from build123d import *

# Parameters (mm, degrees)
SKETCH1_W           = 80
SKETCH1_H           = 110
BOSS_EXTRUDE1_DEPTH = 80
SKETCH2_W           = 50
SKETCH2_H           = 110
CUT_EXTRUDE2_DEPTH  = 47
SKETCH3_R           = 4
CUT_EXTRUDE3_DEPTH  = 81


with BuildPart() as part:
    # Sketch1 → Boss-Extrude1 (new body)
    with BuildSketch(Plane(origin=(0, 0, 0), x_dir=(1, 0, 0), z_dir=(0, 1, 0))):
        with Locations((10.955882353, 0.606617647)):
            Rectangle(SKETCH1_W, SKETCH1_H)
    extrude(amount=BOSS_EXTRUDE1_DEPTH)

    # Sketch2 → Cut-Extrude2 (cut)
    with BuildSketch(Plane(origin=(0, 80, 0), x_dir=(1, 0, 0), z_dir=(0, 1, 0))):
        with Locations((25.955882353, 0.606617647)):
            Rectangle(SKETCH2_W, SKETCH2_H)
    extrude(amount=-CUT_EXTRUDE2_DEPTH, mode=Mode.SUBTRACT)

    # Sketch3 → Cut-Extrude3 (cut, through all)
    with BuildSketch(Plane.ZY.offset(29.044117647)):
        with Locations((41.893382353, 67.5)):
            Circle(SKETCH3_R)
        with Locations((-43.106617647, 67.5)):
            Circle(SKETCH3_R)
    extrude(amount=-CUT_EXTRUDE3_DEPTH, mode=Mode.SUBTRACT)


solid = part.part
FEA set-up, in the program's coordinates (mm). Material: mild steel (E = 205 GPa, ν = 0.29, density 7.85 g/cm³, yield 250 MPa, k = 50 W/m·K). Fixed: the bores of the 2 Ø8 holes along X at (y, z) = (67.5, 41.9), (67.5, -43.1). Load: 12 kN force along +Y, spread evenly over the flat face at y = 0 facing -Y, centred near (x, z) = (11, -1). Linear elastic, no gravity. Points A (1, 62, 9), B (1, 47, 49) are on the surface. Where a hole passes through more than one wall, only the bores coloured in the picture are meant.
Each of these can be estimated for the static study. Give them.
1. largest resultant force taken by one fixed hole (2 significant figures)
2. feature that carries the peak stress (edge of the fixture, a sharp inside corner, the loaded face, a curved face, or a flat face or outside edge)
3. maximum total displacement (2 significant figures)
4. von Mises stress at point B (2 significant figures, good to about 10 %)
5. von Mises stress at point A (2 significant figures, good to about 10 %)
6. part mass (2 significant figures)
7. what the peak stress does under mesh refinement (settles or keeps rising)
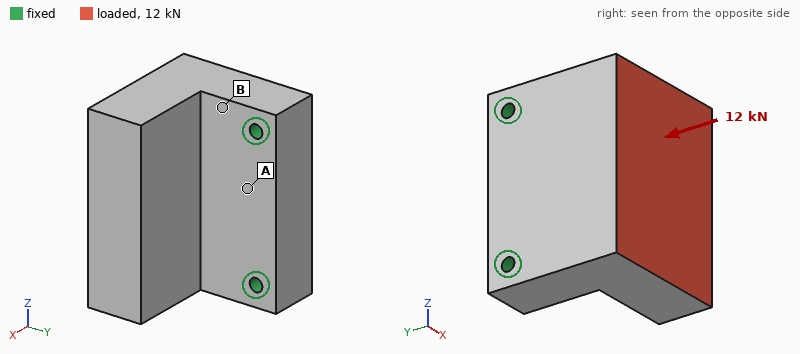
6.2 kN
edge of the fixture
34 µm
28 MPa
7.2 MPa
3.5 kg
keeps rising
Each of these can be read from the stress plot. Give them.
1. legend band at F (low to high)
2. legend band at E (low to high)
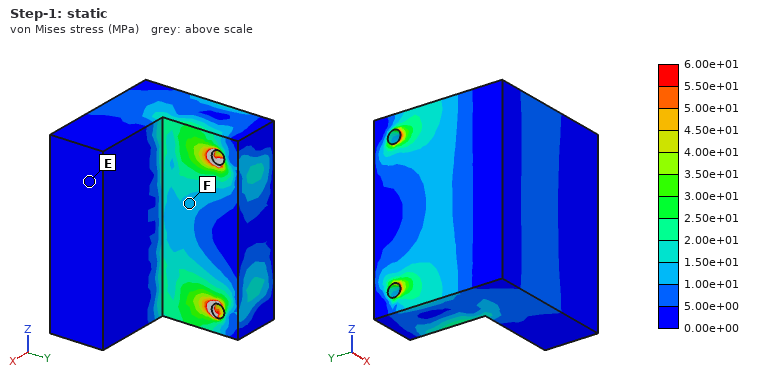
1.00e+01 to 1.50e+01 MPa
0.00e+00 to 5.00e+00 MPa
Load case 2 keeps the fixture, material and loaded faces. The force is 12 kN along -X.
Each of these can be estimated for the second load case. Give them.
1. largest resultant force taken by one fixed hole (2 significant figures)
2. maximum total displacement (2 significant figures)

6.0 kN
68 µm
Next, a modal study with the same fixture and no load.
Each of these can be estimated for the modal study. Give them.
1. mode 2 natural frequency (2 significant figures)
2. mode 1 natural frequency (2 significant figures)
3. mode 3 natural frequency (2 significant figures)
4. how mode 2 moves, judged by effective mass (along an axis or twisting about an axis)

3500 Hz
1800 Hz
5500 Hz
along Z
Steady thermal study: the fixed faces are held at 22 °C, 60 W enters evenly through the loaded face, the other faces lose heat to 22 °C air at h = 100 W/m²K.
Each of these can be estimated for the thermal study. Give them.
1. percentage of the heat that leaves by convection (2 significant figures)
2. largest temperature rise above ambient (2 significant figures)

50 %
17 K
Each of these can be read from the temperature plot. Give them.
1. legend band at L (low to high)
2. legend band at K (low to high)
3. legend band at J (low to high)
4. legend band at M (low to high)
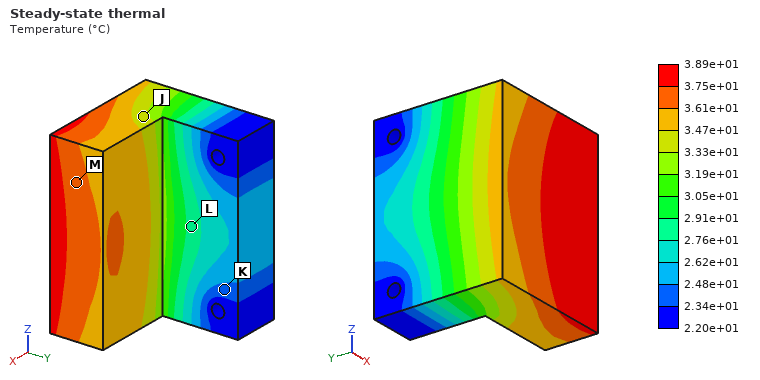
2.76e+01 to 2.91e+01 °C
2.34e+01 to 2.48e+01 °C
3.33e+01 to 3.47e+01 °C
3.61e+01 to 3.75e+01 °C
